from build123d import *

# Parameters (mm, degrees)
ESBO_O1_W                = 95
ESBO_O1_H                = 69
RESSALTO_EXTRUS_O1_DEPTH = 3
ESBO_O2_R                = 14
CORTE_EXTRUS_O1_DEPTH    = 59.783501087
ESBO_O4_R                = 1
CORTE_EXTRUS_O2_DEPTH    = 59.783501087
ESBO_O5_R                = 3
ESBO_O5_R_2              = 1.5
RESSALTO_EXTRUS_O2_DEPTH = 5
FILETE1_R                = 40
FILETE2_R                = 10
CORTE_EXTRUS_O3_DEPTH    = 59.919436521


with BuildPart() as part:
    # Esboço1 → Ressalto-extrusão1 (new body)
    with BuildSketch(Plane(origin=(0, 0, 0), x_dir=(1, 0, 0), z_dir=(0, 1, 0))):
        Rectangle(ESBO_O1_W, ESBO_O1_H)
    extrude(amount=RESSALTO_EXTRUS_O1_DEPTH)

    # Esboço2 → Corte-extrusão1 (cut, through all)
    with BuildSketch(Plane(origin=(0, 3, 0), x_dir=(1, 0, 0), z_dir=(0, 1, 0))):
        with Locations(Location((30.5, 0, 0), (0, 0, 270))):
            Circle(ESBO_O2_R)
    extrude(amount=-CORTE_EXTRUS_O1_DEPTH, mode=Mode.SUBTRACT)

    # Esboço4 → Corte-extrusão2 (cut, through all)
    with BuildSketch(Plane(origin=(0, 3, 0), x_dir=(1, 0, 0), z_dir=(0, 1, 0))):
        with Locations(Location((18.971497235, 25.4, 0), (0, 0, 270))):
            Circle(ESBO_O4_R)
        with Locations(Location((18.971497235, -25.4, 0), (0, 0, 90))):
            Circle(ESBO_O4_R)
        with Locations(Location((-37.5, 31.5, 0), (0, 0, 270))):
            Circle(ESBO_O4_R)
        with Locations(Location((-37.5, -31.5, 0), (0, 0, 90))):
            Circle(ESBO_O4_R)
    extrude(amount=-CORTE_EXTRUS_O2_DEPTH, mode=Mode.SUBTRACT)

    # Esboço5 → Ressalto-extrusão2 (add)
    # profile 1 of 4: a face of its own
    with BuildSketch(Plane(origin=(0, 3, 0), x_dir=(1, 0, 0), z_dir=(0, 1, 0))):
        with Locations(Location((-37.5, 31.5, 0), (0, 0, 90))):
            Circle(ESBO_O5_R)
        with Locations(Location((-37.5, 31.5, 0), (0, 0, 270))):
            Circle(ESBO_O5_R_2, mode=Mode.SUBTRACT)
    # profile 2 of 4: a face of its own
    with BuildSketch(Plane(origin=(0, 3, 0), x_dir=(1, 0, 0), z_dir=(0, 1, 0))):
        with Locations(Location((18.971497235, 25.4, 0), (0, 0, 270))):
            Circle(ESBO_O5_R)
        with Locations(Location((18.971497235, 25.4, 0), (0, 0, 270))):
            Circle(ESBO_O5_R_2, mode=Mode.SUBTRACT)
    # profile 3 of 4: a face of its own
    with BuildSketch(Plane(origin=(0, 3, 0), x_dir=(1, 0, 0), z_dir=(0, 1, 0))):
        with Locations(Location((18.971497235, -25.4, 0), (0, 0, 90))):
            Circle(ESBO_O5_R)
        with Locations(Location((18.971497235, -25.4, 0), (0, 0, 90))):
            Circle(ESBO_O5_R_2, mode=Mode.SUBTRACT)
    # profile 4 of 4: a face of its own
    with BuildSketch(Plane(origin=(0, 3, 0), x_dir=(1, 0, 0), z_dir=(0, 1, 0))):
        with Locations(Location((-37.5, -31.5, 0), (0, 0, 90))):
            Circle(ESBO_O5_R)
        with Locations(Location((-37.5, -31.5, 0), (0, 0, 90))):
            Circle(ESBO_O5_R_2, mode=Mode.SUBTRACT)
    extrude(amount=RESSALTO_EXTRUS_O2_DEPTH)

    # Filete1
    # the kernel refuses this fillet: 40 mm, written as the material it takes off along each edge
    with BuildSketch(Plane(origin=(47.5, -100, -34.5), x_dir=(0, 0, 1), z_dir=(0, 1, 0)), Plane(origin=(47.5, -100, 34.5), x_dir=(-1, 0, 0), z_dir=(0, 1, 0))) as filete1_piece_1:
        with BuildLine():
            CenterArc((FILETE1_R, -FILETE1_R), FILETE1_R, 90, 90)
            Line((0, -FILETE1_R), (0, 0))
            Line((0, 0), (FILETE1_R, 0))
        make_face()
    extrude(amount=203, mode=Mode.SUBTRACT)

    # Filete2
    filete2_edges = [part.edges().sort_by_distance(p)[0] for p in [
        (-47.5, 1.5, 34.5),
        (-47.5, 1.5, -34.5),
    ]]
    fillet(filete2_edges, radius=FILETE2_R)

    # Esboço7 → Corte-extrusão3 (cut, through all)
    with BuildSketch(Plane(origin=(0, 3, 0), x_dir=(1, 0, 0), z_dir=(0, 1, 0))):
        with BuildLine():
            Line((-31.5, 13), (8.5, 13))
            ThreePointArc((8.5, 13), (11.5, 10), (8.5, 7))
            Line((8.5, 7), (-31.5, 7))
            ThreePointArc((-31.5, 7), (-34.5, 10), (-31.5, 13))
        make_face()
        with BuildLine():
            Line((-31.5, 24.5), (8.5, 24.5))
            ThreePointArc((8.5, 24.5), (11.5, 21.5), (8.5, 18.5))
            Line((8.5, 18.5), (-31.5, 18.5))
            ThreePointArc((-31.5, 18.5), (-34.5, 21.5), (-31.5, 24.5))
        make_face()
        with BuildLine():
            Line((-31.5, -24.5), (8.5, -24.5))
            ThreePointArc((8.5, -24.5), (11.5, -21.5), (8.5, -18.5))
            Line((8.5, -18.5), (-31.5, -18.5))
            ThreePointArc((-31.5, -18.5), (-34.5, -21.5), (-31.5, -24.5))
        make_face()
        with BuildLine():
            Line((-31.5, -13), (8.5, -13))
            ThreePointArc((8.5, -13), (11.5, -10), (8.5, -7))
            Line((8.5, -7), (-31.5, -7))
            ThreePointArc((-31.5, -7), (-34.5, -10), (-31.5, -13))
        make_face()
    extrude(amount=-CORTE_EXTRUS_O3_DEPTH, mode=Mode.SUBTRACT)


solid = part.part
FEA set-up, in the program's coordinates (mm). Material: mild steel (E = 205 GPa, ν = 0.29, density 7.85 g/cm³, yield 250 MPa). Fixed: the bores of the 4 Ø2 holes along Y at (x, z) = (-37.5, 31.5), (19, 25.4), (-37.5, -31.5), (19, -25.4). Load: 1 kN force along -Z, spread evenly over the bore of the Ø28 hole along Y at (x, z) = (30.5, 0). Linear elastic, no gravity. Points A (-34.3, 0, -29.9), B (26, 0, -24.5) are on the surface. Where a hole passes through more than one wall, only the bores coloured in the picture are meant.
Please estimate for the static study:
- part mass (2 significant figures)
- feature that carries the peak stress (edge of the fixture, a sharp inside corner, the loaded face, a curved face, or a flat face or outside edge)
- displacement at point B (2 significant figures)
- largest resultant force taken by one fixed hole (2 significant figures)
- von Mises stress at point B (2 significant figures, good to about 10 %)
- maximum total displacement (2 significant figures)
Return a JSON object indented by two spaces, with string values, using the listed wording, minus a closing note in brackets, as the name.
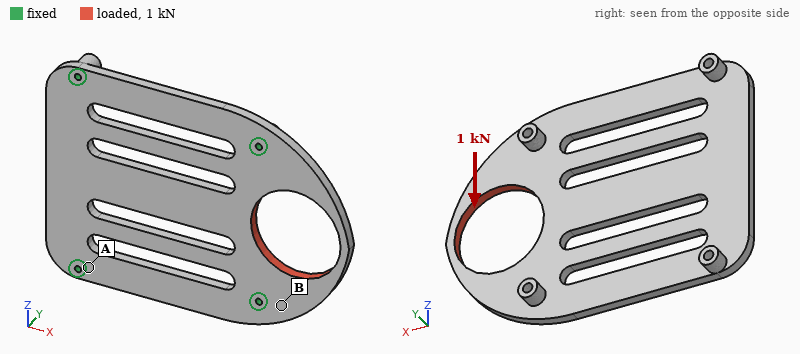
{
  "part mass": "100 g",
  "feature that carries the peak stress": "edge of the fixture",
  "displacement at point B": "1.7 µm",
  "largest resultant force taken by one fixed hole": "530 N",
  "von Mises stress at point B": "14 MPa",
  "maximum total displacement": "11 µm"
}
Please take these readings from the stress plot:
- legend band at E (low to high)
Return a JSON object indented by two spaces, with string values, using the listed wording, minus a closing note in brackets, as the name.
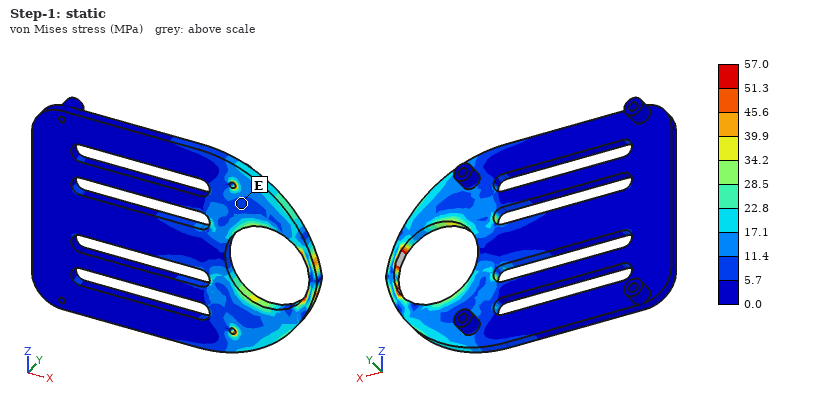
{
  "legend band at E": "5.7 to 11.4 MPa"
}
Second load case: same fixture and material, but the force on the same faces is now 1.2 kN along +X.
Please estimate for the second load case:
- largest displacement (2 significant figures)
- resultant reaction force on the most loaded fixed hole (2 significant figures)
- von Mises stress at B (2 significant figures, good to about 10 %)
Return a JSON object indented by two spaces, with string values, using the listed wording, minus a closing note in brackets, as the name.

{
  "largest displacement": "4.5 µm",
  "resultant reaction force on the most loaded fixed hole": "540 N",
  "von Mises stress at B": "14 MPa"
}
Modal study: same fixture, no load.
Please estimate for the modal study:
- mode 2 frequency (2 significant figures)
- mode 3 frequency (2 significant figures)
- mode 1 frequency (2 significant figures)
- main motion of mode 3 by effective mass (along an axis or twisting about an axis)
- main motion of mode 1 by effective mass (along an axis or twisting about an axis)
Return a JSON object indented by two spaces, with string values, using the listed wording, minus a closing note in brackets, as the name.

{
  "mode 2 frequency": "3500 Hz",
  "mode 3 frequency": "4100 Hz",
  "mode 1 frequency": "2500 Hz",
  "main motion of mode 3 by effective mass": "twisting about Z",
  "main motion of mode 1 by effective mass": "along Y"
}
